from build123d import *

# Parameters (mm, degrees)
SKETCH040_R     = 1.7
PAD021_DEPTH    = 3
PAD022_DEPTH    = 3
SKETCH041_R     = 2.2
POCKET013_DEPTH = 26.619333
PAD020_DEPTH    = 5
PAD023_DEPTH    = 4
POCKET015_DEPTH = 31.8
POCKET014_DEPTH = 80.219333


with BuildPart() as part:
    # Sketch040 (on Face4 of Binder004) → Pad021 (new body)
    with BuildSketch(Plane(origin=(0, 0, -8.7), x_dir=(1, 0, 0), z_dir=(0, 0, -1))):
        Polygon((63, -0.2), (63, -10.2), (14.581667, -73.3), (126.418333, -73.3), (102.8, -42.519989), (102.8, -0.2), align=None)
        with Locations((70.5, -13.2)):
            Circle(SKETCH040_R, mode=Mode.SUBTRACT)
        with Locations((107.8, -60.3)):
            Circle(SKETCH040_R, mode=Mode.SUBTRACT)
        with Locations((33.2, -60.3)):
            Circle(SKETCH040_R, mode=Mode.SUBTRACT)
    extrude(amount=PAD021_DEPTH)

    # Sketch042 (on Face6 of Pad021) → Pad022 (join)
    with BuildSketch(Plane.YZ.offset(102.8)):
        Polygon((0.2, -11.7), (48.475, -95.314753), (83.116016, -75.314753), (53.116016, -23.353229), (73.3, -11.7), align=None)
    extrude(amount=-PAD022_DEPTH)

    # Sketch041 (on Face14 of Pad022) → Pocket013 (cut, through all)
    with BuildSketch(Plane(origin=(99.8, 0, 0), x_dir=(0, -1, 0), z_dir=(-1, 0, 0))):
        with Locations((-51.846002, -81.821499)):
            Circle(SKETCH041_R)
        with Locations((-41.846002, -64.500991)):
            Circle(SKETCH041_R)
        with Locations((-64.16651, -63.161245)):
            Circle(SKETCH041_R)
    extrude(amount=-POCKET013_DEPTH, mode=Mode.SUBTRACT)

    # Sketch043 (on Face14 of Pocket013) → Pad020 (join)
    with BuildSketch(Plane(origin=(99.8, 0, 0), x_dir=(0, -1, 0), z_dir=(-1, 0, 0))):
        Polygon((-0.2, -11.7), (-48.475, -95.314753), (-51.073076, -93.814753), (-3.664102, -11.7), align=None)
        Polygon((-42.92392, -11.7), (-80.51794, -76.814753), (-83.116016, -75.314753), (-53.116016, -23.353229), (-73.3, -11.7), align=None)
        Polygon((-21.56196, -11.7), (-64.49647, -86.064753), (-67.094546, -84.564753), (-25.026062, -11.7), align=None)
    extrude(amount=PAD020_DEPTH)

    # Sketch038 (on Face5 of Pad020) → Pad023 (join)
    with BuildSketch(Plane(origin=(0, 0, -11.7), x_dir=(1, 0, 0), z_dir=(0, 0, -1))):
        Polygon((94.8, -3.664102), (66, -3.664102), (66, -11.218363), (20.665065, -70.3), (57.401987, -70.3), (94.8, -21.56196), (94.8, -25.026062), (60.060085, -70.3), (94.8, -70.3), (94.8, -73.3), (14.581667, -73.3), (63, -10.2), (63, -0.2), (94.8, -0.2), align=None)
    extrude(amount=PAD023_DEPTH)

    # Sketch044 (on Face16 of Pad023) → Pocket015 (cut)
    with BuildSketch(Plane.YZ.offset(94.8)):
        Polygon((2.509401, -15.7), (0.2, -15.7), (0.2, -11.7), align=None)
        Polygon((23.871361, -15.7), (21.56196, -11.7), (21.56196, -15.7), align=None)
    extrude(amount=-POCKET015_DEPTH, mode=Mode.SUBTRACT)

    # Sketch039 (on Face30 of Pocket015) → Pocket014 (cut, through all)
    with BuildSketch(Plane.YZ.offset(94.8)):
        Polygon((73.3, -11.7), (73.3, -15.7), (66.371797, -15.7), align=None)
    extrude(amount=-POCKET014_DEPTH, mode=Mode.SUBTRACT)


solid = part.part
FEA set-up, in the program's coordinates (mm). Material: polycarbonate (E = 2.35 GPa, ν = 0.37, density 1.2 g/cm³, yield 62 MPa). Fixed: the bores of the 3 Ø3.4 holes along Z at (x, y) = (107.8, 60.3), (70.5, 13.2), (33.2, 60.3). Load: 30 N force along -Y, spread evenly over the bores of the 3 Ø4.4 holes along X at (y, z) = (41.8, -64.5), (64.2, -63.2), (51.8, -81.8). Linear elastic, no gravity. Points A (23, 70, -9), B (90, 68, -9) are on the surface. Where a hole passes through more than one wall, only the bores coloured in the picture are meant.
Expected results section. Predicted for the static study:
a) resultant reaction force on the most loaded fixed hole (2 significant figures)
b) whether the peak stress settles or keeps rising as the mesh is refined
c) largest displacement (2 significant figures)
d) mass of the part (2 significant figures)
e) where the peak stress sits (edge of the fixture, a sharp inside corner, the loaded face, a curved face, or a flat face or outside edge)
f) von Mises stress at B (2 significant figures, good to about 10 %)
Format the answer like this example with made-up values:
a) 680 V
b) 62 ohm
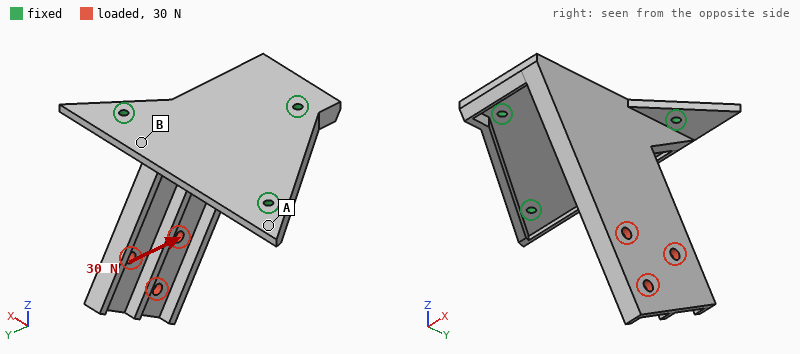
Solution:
a) 30 N
b) keeps rising
c) 1.7 mm
d) 38 g
e) edge of the fixture
f) 2.3 MPa
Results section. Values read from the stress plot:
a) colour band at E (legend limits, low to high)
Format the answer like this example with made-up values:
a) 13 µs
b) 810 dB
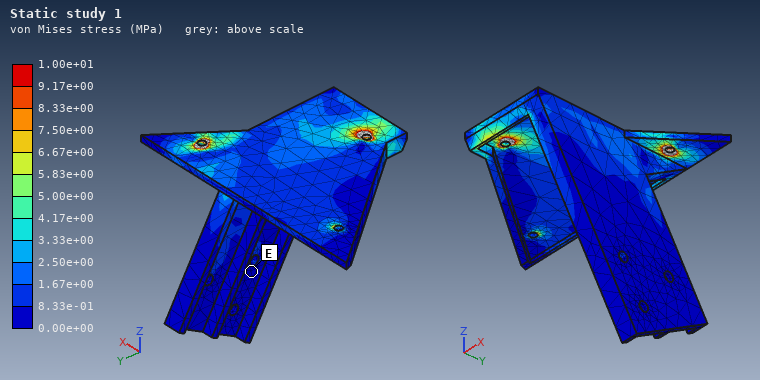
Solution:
a) 0.00e+00 to 8.33e-01 MPa
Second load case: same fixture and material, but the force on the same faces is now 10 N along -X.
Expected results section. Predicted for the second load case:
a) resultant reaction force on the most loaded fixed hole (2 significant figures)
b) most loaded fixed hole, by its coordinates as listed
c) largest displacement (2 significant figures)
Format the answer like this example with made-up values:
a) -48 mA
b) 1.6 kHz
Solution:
a) 13 N
b) (107.8, 60.3)
c) 1.8 mm
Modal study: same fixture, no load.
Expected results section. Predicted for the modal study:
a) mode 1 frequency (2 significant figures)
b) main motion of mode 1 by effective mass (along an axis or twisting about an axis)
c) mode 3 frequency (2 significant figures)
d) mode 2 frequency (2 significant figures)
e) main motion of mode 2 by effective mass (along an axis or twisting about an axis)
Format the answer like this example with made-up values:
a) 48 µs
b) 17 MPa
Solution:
a) 160 Hz
b) along X
c) 510 Hz
d) 340 Hz
e) along Y
